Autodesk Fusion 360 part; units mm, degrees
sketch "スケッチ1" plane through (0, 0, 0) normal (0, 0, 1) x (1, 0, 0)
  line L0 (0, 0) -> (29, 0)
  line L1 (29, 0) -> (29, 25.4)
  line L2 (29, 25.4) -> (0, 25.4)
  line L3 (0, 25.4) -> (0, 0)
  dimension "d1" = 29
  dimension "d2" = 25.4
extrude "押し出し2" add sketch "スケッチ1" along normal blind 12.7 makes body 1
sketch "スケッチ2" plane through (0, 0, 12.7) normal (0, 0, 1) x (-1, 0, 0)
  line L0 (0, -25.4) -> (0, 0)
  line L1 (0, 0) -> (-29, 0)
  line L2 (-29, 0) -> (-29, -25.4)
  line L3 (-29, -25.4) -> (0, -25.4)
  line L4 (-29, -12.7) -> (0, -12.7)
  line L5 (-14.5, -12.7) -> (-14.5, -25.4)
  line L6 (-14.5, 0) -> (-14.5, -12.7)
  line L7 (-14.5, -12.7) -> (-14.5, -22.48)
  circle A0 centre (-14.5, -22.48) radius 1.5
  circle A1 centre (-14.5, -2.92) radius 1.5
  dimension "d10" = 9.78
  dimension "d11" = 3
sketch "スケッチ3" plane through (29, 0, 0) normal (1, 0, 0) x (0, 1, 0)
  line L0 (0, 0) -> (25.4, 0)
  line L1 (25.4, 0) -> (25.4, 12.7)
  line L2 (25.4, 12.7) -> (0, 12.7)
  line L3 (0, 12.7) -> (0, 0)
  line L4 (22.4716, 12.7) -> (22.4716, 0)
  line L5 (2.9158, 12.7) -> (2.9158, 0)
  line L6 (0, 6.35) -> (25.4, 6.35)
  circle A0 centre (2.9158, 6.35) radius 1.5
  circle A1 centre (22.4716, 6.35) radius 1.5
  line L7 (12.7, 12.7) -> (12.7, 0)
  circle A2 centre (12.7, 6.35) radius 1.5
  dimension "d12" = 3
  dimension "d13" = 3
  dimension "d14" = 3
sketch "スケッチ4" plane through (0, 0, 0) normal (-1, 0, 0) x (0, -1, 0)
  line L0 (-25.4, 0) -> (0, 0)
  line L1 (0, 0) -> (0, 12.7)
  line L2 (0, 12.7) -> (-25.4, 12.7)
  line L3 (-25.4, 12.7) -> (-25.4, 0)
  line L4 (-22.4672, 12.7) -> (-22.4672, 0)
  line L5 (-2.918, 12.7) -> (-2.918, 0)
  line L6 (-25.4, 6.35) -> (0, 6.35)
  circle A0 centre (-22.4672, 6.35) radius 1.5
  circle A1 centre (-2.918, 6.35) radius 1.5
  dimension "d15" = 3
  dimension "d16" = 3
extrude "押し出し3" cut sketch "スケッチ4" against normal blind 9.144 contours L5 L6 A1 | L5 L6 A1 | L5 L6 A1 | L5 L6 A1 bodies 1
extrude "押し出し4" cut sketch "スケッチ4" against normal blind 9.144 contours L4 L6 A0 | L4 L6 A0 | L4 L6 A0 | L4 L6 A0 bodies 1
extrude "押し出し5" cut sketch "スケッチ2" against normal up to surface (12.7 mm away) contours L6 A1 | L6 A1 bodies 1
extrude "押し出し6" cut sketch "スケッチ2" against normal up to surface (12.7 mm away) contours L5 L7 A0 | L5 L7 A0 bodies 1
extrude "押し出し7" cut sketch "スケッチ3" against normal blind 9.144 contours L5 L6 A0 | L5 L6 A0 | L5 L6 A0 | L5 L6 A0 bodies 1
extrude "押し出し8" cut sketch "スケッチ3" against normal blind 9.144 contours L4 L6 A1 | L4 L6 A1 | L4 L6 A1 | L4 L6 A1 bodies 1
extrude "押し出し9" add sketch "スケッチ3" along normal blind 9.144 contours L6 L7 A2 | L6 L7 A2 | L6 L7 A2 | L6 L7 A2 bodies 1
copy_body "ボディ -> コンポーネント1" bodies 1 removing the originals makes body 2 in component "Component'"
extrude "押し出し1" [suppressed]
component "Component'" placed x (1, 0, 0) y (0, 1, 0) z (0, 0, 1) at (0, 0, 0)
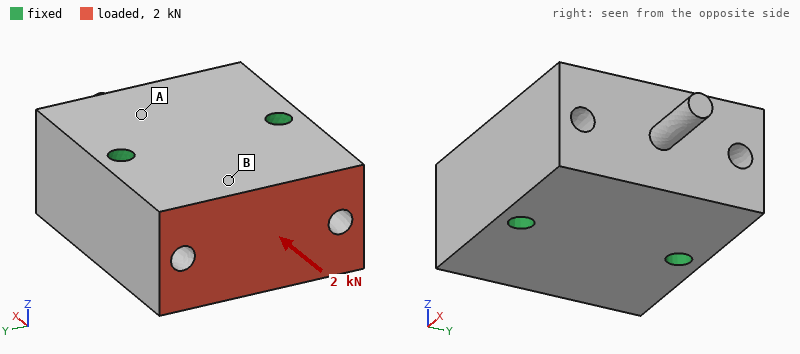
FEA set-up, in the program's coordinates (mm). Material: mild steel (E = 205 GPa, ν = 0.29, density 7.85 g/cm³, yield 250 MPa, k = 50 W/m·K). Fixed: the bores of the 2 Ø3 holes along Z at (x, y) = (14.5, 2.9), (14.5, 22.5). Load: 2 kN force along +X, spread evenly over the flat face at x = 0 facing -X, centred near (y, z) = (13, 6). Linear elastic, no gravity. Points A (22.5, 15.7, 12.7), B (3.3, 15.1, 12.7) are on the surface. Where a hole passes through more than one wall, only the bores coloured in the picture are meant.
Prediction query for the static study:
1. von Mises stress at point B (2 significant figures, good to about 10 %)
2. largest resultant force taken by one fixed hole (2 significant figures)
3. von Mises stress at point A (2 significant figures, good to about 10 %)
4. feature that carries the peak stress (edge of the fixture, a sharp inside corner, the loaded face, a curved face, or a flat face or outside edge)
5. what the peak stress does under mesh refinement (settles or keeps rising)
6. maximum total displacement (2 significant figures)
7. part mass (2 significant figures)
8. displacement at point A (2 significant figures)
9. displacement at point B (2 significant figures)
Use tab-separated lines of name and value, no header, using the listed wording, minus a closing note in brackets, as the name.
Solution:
von Mises stress at point B	5.7 MPa
largest resultant force taken by one fixed hole	1.0 kN
von Mises stress at point A	1.8 MPa
feature that carries the peak stress	edge of the fixture
what the peak stress does under mesh refinement	keeps rising
maximum total displacement	0.57 µm
part mass	71 g
displacement at point A	0.16 µm
displacement at point B	0.47 µm
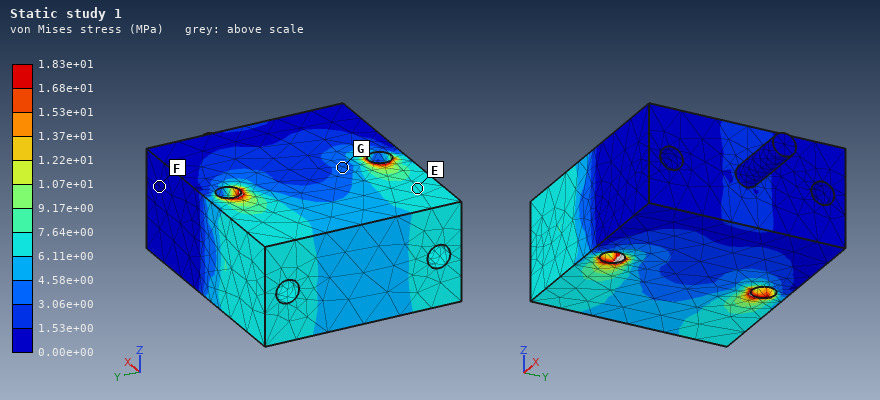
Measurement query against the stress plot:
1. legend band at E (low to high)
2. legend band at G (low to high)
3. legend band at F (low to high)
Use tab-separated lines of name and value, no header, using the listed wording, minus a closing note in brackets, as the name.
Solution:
legend band at E	6.11e+00 to 7.64e+00 MPa
legend band at G	3.06e+00 to 4.58e+00 MPa
legend band at F	0.00e+00 to 1.53e+00 MPa
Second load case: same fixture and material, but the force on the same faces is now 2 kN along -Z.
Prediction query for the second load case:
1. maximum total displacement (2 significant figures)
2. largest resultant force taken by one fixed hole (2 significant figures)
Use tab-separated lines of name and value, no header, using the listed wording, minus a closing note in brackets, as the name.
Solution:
maximum total displacement	5.4 µm
largest resultant force taken by one fixed hole	1.0 kN
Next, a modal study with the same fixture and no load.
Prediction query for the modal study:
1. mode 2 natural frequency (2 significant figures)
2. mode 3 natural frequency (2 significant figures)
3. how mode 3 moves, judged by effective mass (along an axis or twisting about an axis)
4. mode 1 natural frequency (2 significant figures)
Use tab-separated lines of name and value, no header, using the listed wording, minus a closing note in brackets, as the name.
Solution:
mode 2 natural frequency	21 kHz
mode 3 natural frequency	28 kHz
how mode 3 moves, judged by effective mass	twisting about Y
mode 1 natural frequency	21 kHz
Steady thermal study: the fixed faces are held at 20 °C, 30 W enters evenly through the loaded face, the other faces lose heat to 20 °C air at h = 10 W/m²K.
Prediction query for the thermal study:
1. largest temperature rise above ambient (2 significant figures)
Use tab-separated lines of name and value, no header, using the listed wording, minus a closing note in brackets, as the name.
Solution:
largest temperature rise above ambient	30 K
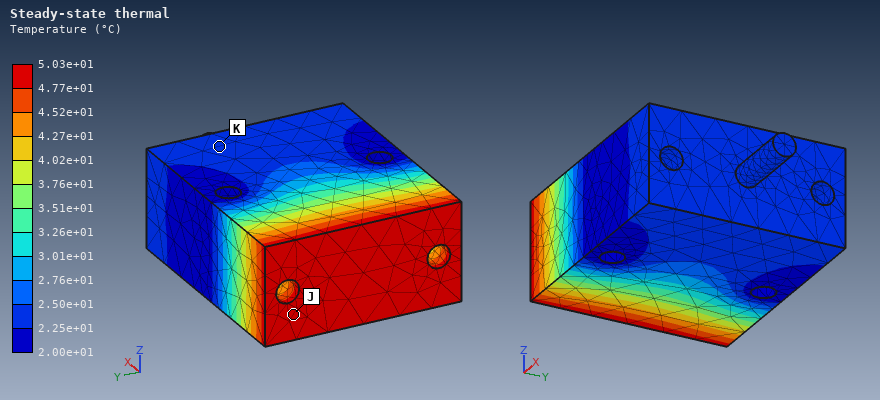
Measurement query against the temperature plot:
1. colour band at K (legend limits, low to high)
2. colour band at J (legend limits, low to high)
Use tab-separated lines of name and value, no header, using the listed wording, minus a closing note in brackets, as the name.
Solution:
colour band at K	2.25e+01 to 2.50e+01 °C
colour band at J	4.77e+01 to 5.03e+01 °C
